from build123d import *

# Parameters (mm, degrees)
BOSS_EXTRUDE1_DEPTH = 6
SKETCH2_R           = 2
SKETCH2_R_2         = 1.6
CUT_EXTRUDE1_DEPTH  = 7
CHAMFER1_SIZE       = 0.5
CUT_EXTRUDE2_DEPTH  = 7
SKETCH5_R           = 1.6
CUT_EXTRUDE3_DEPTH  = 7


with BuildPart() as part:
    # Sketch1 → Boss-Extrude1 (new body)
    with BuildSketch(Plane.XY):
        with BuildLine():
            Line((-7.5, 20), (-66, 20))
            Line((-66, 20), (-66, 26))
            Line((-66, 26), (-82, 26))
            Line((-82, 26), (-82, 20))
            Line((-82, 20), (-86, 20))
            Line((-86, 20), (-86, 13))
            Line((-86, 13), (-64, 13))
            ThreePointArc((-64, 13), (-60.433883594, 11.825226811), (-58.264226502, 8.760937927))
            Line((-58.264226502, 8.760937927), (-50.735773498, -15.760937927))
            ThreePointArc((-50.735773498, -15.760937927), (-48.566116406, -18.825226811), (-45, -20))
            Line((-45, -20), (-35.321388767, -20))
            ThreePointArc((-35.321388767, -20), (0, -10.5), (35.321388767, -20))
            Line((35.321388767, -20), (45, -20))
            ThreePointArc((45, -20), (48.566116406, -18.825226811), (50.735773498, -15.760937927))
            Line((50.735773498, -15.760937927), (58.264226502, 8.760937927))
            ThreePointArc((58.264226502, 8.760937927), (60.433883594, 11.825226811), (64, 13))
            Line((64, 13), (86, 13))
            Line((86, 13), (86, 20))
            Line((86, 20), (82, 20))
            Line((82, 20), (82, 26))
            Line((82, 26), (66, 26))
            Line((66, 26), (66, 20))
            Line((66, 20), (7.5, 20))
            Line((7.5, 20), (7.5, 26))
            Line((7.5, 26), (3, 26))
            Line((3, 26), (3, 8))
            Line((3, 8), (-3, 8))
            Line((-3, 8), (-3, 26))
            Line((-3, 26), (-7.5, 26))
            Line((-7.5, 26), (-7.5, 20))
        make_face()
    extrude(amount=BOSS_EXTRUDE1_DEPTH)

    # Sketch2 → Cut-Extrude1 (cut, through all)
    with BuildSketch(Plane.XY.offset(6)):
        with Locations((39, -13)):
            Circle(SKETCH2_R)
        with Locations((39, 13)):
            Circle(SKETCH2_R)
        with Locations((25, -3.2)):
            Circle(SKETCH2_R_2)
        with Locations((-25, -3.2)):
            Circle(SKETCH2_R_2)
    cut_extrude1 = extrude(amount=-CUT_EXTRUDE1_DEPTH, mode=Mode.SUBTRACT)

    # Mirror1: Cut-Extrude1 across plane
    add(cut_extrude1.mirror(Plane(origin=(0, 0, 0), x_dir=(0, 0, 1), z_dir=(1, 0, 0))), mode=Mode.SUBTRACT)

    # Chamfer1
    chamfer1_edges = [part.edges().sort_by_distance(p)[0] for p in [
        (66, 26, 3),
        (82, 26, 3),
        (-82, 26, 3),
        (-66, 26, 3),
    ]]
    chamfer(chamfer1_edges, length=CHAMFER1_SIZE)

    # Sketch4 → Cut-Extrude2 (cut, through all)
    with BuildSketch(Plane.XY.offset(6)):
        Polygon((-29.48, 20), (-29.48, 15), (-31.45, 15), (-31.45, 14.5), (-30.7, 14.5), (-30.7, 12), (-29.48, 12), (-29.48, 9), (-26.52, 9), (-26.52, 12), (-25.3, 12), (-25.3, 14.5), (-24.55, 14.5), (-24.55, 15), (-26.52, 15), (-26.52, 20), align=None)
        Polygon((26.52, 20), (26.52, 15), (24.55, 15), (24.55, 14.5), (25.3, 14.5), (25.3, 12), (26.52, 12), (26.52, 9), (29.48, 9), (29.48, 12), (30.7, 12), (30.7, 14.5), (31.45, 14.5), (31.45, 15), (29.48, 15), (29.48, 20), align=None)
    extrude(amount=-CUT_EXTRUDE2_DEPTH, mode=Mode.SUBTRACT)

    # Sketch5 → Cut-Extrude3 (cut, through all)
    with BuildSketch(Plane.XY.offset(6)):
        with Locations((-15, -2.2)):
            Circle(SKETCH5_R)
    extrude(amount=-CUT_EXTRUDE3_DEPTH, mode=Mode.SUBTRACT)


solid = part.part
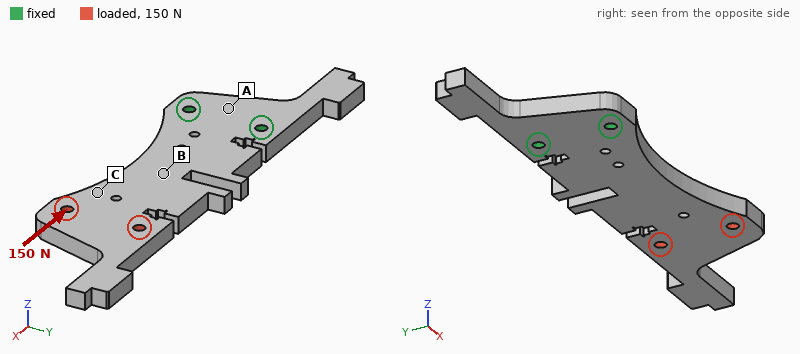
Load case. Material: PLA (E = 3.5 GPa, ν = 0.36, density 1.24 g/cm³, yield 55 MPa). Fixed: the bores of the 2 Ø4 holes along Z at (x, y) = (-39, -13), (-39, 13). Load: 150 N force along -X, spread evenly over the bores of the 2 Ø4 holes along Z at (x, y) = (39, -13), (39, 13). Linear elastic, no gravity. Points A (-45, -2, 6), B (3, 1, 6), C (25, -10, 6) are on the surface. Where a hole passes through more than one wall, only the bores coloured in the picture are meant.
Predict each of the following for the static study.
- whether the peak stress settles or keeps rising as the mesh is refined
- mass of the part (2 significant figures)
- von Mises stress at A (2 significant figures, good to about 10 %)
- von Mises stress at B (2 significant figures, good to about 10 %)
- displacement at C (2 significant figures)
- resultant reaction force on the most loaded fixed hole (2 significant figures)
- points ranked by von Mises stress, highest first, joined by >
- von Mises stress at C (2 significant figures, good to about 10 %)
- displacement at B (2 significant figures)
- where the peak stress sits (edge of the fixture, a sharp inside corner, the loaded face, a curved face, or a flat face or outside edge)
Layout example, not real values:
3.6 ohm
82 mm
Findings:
keeps rising
32 g
0.35 MPa
1.2 MPa
27 µm
78 N
B > C > A
0.70 MPa
20 µm
a sharp inside corner
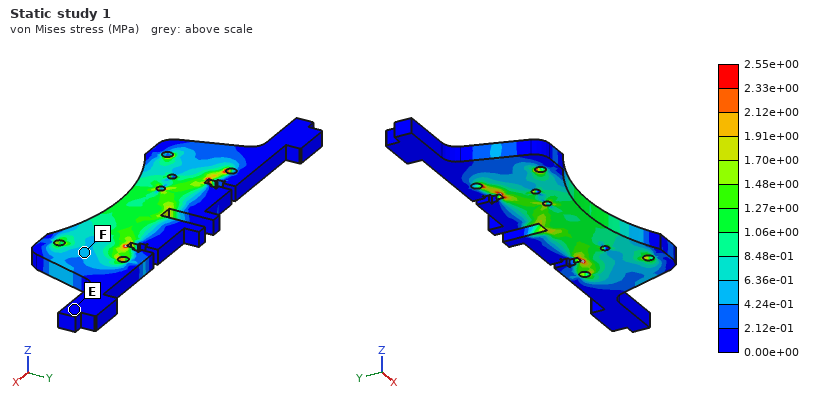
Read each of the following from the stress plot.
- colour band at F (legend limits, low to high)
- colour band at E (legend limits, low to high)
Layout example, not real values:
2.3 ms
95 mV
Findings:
4.24e-01 to 6.36e-01 MPa
0.00e+00 to 2.12e-01 MPa
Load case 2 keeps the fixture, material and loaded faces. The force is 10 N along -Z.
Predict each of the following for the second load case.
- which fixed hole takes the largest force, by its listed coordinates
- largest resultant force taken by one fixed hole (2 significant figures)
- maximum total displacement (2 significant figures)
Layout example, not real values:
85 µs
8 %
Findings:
(-39, -13)
6.0 N
2.0 mm
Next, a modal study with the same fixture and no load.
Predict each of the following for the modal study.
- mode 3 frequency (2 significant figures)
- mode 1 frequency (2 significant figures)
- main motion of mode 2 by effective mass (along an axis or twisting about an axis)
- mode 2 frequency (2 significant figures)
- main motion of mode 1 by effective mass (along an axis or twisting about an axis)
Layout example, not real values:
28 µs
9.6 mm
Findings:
560 Hz
120 Hz
along Y
440 Hz
along Z
